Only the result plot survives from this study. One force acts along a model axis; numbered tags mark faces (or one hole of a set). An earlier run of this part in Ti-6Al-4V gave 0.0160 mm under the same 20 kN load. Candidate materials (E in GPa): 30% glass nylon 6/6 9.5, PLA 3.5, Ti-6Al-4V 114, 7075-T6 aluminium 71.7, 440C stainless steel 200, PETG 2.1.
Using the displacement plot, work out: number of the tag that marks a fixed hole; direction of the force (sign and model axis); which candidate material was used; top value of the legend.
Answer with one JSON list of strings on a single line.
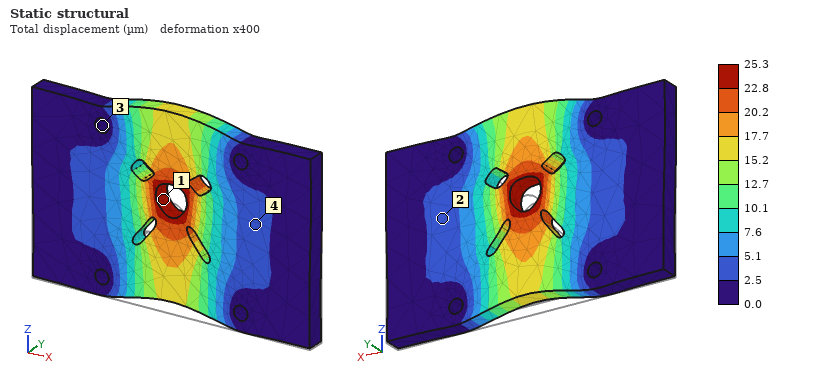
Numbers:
["3", "+Z", "7075-T6 aluminium", "25.3 µm"]
